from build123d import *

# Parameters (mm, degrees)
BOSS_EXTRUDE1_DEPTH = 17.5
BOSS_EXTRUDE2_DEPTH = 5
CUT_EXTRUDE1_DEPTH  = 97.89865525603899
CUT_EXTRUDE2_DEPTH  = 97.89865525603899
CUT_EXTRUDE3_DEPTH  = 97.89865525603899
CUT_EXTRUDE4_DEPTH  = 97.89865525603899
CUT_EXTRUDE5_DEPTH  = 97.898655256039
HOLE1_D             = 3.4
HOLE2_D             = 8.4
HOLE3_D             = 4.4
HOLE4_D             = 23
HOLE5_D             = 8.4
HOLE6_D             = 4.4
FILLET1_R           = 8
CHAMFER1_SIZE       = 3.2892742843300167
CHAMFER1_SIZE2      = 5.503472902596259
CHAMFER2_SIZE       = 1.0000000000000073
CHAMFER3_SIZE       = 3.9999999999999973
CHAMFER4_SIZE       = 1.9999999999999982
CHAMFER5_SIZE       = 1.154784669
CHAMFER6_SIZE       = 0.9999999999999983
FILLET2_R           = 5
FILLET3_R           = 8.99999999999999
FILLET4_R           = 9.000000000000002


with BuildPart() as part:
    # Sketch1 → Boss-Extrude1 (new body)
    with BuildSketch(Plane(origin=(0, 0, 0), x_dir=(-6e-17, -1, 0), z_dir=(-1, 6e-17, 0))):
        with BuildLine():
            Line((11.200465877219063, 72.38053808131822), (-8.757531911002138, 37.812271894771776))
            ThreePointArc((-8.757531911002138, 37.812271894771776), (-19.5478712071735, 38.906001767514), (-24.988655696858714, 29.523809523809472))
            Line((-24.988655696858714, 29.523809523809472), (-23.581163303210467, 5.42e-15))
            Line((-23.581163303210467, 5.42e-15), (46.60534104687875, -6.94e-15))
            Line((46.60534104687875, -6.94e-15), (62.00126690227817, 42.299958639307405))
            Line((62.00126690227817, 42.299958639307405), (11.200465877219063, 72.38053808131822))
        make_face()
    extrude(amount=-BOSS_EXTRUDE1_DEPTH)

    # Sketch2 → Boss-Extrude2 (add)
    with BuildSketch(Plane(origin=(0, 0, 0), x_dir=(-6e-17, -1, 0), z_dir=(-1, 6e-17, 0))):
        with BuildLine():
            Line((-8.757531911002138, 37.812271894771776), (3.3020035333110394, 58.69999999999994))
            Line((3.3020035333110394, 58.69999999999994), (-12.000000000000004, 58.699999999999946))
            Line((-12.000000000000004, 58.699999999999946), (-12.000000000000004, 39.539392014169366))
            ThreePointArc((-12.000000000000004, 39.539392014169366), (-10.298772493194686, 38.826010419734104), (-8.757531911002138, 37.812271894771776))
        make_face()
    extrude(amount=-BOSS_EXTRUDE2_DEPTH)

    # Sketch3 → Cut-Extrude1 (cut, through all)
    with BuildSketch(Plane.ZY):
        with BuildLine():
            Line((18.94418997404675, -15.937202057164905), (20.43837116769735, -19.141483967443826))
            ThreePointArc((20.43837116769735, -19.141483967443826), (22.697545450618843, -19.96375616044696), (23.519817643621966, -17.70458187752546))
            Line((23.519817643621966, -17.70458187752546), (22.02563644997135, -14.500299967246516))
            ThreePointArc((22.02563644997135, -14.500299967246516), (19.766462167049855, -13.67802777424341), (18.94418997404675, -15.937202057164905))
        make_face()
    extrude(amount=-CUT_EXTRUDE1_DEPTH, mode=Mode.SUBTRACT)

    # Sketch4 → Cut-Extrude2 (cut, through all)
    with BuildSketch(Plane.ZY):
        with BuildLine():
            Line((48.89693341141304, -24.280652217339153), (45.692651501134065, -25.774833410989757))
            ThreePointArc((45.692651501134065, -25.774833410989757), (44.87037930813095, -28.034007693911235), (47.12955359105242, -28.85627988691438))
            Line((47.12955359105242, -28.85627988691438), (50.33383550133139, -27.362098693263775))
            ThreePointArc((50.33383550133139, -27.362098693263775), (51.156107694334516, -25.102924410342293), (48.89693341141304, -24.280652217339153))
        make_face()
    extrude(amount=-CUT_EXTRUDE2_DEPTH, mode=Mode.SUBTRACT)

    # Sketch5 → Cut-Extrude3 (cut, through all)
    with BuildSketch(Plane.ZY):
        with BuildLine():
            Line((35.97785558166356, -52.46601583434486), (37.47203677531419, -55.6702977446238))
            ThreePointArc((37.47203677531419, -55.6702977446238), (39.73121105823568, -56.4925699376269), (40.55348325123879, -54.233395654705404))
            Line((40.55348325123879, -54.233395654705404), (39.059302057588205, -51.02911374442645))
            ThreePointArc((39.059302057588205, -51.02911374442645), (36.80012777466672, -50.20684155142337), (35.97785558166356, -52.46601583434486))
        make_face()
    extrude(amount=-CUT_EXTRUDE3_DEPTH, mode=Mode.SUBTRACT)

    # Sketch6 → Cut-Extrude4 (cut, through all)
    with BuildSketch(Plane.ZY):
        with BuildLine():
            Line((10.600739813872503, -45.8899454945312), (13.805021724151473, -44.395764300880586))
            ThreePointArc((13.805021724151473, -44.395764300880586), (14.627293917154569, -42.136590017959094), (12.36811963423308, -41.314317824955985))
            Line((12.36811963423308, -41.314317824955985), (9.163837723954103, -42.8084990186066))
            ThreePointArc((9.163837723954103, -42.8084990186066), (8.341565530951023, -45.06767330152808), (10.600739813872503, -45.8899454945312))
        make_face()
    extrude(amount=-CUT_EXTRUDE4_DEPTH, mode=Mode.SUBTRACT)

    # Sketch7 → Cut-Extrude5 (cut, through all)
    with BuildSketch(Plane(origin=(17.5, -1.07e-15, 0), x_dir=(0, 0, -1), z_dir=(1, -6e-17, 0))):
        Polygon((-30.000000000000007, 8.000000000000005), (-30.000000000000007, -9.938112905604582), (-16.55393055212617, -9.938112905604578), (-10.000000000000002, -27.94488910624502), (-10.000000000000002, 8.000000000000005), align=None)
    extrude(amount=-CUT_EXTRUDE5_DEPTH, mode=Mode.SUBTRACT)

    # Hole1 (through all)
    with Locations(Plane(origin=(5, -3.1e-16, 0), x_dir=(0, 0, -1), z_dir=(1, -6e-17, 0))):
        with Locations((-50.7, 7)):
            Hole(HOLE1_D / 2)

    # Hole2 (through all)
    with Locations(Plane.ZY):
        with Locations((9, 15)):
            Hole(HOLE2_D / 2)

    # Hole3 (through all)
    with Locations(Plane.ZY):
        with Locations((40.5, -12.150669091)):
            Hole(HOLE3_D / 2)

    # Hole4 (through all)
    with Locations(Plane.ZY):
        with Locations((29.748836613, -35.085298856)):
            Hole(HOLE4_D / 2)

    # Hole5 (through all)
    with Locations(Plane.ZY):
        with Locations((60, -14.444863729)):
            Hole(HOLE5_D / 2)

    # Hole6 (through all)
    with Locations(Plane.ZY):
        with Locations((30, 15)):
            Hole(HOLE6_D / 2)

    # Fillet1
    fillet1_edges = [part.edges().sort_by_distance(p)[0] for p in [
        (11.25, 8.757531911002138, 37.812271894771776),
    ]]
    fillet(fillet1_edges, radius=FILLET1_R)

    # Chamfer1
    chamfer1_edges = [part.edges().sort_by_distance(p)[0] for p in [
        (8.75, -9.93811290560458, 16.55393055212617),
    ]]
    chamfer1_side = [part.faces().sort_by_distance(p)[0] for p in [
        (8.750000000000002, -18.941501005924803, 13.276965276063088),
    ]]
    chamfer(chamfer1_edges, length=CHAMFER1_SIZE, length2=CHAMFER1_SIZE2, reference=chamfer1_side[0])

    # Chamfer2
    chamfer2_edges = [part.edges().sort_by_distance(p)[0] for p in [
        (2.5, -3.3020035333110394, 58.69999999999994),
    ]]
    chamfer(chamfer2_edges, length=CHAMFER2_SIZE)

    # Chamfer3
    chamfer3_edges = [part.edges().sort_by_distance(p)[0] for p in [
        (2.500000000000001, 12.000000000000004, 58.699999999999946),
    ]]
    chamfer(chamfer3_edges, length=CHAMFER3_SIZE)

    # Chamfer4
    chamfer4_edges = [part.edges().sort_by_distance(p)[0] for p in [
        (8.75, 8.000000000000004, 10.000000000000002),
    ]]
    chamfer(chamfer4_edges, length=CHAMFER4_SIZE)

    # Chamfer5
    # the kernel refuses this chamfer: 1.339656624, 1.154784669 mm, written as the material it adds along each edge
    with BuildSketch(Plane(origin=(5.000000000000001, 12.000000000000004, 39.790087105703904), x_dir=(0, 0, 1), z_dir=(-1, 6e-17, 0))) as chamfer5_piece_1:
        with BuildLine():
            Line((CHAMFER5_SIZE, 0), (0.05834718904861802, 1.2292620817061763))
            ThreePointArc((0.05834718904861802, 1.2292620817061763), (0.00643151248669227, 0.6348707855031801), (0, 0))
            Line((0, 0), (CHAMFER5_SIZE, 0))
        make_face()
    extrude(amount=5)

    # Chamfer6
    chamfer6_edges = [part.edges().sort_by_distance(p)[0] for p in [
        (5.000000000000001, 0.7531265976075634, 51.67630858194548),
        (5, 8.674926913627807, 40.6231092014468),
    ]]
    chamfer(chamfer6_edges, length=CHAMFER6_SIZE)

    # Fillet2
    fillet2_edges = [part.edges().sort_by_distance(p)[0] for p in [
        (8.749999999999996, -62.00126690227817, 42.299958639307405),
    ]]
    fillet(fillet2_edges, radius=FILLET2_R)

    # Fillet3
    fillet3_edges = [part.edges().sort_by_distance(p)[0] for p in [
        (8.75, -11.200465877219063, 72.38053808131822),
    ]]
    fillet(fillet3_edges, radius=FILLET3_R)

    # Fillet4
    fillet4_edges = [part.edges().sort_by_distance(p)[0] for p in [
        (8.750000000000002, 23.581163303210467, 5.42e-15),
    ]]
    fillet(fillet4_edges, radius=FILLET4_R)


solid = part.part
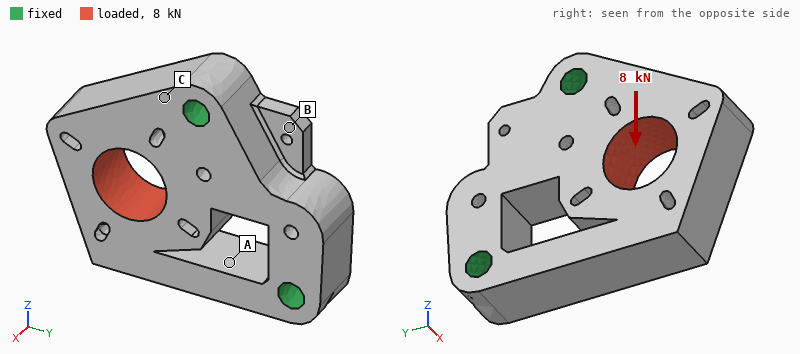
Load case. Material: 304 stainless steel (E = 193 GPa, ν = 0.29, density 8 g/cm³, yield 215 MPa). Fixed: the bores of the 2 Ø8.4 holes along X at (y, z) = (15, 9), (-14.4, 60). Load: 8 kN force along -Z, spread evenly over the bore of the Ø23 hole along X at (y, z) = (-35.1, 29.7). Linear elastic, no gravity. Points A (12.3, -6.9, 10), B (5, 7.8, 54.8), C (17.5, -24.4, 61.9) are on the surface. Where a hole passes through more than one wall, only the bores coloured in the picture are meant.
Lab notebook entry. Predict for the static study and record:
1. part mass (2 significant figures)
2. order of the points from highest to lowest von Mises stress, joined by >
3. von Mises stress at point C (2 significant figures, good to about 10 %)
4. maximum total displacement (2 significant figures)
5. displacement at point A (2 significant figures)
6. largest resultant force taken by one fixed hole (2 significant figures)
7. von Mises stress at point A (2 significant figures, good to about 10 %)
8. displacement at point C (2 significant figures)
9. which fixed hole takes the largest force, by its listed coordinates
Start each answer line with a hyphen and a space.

- 450 g
- C > A > B
- 22 MPa
- 10 µm
- 3.0 µm
- 8.2 kN
- 12 MPa
- 1.9 µm
- (-14.4, 60)
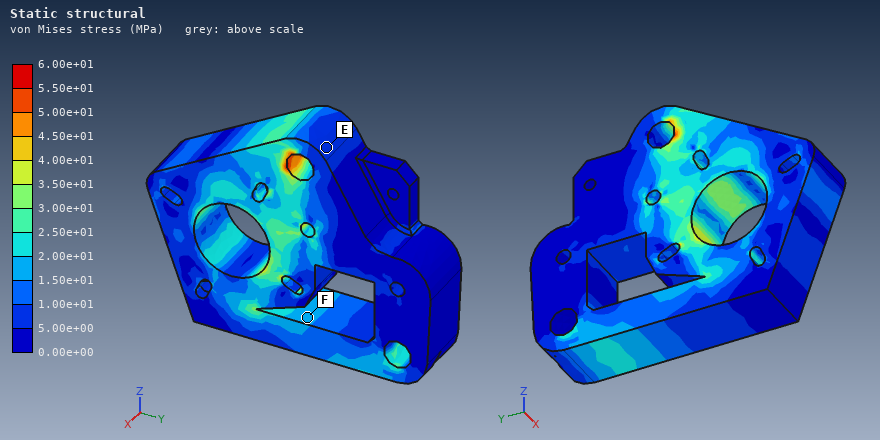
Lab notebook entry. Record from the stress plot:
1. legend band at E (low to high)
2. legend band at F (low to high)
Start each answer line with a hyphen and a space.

- 5.00e+00 to 1.00e+01 MPa
- 1.50e+01 to 2.00e+01 MPa
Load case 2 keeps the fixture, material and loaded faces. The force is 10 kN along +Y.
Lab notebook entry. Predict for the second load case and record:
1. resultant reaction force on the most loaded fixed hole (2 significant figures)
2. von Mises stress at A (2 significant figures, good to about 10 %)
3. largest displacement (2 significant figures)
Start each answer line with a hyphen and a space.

- 5.2 kN
- 30 MPa
- 9.3 µm
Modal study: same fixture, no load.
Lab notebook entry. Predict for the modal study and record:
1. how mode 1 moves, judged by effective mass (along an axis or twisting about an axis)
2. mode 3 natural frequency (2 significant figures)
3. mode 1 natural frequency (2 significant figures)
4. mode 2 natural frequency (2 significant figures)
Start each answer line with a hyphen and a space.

- along X
- 9500 Hz
- 4000 Hz
- 8700 Hz
